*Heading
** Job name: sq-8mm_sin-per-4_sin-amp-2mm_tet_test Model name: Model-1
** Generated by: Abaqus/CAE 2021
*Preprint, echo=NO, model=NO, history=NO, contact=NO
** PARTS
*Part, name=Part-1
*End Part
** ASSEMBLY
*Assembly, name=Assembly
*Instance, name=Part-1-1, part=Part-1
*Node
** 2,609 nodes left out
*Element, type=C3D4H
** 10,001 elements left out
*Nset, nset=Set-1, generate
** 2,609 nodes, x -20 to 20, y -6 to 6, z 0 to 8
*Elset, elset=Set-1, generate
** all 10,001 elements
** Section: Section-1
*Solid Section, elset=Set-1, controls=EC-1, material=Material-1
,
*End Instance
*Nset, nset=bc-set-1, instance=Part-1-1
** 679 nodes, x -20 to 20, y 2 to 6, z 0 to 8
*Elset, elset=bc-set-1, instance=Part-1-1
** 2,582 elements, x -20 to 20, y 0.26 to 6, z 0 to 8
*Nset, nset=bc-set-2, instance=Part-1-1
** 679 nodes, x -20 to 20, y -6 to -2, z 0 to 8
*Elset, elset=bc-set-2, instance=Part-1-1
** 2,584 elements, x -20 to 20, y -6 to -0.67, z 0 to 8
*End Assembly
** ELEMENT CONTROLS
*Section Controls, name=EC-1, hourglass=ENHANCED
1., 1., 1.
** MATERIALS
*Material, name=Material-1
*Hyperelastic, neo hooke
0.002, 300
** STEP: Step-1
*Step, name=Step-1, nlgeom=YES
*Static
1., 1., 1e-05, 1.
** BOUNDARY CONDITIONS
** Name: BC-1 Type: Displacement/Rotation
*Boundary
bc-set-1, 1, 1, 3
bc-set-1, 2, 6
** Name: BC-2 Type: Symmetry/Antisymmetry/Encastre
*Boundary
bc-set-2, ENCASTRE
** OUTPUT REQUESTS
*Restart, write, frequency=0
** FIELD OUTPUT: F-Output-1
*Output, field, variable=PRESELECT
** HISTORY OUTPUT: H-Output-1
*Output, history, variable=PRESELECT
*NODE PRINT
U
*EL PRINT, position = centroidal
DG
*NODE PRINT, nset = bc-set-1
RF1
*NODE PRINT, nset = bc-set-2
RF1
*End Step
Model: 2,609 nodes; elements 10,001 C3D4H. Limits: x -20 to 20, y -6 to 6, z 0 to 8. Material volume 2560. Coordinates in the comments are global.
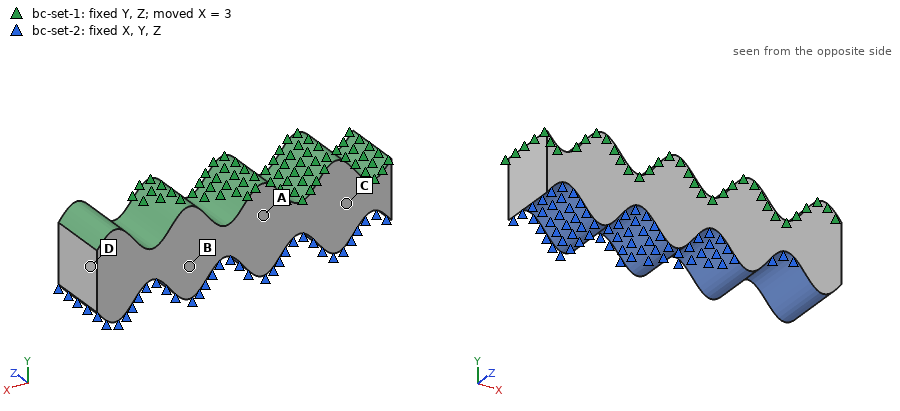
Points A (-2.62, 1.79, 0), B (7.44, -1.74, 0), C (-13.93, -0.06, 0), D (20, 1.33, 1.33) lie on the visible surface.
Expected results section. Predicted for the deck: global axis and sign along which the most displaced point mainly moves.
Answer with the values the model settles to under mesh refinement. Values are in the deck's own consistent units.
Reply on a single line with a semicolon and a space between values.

+X
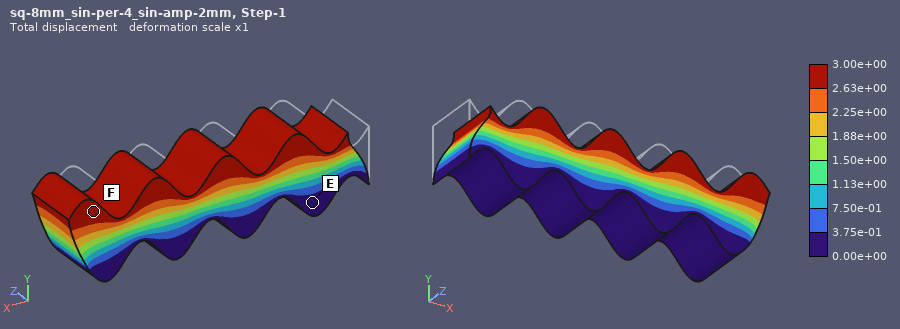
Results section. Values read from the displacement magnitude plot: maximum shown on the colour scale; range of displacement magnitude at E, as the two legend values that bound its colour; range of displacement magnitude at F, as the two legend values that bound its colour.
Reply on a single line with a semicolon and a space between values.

3.00e+00; 0.00e+00 to 3.75e-01; 2.63e+00 to 3.00e+00
